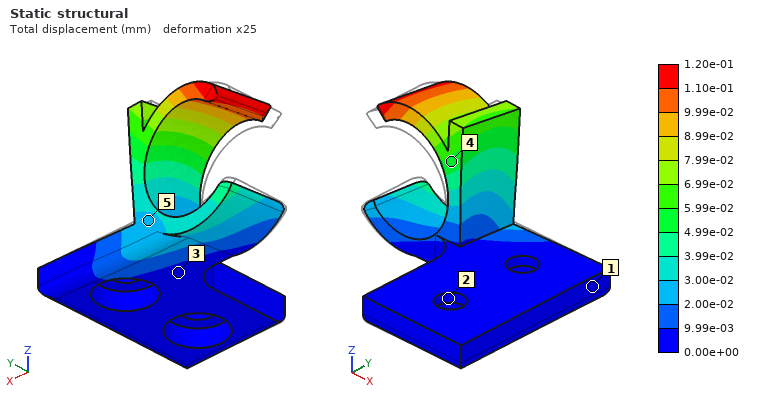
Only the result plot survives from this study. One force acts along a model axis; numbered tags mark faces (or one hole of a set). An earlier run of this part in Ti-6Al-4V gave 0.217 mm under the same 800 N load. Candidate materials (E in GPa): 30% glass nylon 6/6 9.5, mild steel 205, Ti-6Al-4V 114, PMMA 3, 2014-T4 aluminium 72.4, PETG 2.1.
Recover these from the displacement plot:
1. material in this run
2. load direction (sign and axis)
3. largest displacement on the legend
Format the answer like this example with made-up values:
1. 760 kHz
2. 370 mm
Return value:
1. mild steel
2. +Y
3. 1.20e-01 mm
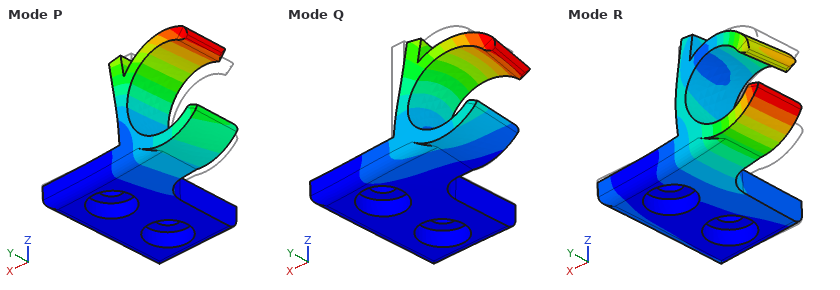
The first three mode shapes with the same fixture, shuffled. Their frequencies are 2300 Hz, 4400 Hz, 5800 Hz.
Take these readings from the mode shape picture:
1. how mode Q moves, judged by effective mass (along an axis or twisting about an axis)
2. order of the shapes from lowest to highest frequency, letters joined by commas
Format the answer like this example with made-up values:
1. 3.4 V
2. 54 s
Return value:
1. along Y
2. P, Q, R
